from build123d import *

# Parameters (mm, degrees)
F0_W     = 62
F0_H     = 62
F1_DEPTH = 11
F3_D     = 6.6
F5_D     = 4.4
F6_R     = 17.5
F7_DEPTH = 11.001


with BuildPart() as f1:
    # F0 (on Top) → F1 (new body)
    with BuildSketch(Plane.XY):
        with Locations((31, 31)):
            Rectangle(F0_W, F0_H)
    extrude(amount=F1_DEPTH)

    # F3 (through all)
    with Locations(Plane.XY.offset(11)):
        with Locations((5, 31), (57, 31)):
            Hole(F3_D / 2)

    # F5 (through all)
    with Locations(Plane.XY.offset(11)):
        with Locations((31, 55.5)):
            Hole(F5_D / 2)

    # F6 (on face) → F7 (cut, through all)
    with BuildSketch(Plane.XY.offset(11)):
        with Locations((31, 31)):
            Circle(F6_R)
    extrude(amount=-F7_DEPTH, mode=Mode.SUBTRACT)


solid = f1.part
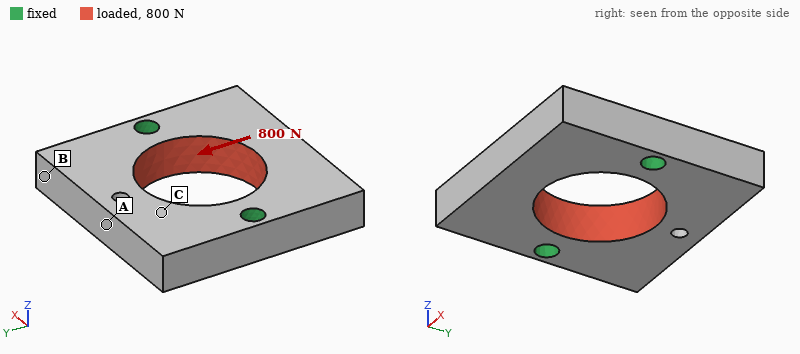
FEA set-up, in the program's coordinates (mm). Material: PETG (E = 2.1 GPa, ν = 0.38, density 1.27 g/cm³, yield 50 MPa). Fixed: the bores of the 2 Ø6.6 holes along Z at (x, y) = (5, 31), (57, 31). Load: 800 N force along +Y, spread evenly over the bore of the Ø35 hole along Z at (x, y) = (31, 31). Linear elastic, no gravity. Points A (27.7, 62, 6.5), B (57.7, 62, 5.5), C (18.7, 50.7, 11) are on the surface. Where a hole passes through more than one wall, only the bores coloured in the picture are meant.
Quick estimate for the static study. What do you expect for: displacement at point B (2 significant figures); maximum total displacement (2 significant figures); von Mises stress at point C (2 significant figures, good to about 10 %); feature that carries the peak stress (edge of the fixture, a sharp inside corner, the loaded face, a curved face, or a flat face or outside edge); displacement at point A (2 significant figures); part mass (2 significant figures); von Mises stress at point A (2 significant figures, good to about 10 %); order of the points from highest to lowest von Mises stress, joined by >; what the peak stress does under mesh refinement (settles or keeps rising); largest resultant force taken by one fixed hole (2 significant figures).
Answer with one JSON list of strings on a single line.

["12 µm", "31 µm", "0.99 MPa", "edge of the fixture", "24 µm", "39 g", "1.9 MPa", "A > C > B", "keeps rising", "400 N"]
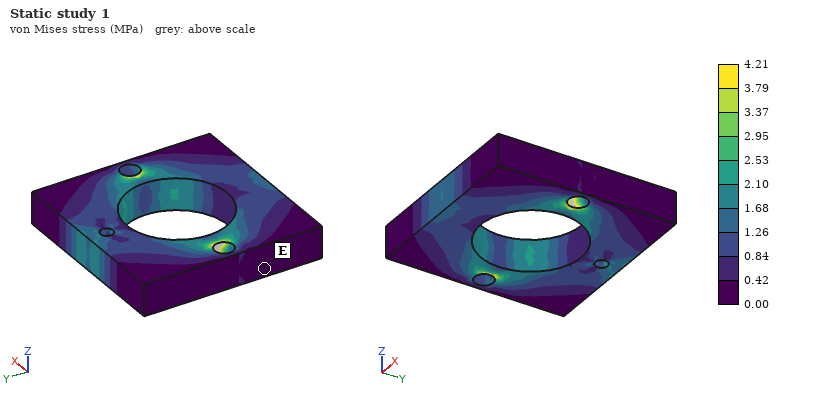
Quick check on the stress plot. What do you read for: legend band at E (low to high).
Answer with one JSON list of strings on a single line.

["0.00 to 0.42 MPa"]
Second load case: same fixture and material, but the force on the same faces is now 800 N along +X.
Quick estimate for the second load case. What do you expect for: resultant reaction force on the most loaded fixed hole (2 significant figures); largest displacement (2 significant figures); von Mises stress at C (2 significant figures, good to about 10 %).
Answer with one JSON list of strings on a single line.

["400 N", "40 µm", "0.60 MPa"]
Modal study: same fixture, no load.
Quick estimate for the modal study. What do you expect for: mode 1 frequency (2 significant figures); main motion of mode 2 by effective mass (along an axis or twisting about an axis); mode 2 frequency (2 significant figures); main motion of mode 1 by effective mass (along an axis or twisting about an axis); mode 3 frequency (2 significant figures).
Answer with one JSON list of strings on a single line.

["1600 Hz", "along Z", "1700 Hz", "twisting about X", "2800 Hz"]
